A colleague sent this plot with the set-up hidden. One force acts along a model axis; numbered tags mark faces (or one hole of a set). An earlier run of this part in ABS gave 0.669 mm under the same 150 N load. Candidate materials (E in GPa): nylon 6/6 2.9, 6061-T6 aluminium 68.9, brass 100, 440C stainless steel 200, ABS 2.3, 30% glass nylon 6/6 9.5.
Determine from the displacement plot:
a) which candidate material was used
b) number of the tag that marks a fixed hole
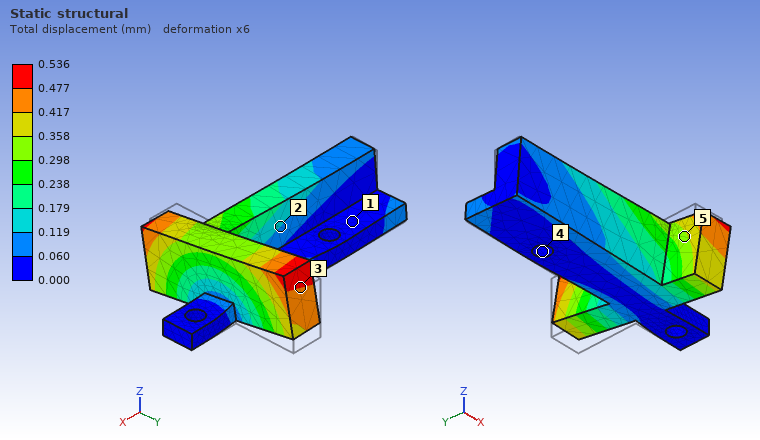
nylon 6/6
4
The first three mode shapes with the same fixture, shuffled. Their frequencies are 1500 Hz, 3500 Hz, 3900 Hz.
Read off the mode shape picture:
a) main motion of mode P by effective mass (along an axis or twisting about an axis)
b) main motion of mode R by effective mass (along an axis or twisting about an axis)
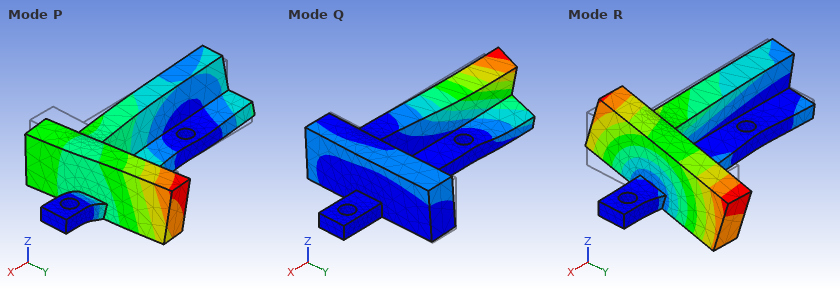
along Z
along Y
